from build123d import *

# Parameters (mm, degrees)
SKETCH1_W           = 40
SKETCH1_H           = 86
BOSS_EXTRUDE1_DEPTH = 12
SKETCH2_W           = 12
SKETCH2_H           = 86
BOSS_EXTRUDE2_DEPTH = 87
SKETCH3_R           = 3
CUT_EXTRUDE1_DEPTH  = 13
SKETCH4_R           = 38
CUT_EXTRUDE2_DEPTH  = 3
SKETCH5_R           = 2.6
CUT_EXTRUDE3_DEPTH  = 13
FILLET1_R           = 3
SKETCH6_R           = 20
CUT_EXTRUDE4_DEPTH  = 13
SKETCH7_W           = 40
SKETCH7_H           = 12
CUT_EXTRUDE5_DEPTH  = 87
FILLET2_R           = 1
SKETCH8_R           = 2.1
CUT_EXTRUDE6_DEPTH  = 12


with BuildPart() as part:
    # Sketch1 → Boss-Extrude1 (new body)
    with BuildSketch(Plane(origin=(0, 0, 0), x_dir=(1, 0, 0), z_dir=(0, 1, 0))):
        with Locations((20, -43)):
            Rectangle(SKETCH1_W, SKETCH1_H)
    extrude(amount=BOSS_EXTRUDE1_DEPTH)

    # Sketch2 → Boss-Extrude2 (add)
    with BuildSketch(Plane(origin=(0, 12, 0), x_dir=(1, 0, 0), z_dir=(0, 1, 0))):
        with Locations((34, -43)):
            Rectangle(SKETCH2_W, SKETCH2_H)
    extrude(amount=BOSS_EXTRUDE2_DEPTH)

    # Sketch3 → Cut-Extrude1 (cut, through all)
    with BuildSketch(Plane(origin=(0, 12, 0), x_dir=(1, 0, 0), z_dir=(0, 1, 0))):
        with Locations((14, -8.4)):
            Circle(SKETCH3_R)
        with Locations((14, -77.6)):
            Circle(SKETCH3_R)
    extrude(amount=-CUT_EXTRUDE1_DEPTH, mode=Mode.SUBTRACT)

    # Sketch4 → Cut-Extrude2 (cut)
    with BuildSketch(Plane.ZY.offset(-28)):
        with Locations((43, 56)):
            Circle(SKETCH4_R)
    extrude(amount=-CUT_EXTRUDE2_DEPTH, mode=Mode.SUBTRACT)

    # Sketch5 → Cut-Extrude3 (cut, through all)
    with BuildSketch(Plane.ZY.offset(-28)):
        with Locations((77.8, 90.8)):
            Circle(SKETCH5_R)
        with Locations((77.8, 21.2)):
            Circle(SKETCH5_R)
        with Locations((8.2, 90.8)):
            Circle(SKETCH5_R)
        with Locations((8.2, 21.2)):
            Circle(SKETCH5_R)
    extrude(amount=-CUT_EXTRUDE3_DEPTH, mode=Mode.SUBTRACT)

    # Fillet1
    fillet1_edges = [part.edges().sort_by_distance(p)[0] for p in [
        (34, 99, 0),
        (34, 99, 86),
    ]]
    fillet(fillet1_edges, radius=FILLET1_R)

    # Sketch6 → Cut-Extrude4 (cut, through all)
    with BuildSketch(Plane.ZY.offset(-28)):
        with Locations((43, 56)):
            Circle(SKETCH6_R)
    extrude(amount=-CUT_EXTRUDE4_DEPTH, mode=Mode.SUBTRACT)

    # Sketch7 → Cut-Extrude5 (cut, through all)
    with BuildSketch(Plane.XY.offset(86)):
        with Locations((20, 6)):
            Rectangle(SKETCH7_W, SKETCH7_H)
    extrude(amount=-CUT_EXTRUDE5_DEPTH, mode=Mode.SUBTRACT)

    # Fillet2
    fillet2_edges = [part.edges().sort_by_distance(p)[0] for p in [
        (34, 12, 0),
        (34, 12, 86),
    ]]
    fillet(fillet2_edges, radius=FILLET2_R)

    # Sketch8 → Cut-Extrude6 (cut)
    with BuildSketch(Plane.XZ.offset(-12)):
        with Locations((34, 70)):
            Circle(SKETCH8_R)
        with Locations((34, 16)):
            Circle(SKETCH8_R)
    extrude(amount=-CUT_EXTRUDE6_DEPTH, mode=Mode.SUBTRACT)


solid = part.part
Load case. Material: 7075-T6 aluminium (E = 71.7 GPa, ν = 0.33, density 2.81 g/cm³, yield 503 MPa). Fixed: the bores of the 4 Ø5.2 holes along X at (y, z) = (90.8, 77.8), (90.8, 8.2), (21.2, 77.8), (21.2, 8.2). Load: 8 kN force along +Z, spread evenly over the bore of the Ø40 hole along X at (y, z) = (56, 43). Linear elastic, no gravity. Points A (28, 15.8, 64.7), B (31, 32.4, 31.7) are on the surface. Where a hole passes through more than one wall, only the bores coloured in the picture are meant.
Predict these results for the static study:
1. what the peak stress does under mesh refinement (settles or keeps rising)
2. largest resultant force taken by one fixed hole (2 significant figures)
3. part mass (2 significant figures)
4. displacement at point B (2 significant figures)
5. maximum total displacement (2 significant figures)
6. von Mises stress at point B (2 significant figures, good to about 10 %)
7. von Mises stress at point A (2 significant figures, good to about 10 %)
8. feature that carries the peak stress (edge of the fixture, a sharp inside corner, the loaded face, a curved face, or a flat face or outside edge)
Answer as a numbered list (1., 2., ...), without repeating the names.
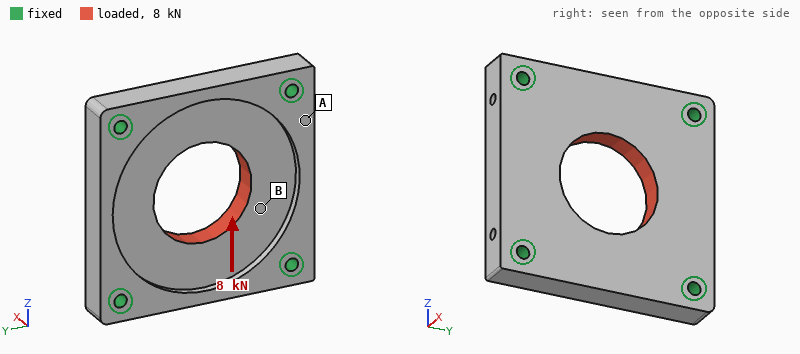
1. keeps rising
2. 2.2 kN
3. 180 g
4. 4.2 µm
5. 8.7 µm
6. 11 MPa
7. 6.6 MPa
8. edge of the fixture
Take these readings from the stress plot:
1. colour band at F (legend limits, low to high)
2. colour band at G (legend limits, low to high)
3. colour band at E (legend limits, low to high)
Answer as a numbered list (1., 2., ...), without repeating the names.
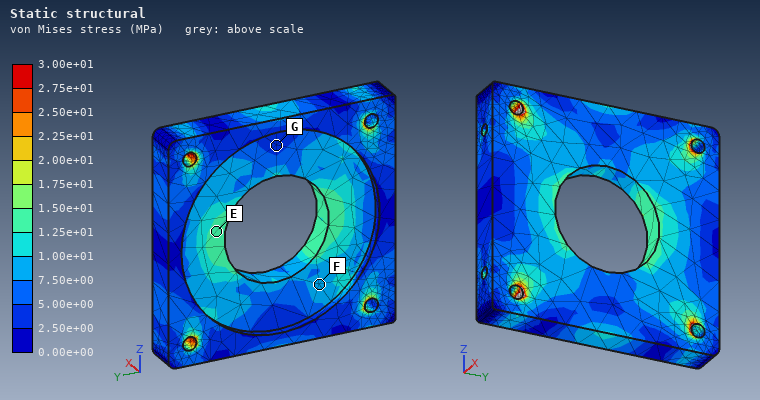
1. 7.50e+00 to 1.00e+01 MPa
2. 2.50e+00 to 5.00e+00 MPa
3. 1.25e+01 to 1.50e+01 MPa
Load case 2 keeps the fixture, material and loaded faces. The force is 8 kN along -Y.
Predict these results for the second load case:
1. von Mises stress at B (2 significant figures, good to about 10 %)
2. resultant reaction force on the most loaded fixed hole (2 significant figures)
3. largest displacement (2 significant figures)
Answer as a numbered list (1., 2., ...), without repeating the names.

1. 7.6 MPa
2. 2.1 kN
3. 8.6 µm
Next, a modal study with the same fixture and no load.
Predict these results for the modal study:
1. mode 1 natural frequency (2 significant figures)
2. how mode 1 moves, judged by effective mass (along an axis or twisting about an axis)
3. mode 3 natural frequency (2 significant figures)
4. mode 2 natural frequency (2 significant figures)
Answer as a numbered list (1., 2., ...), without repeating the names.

1. 8400 Hz
2. along X
3. 11 kHz
4. 10 kHz
